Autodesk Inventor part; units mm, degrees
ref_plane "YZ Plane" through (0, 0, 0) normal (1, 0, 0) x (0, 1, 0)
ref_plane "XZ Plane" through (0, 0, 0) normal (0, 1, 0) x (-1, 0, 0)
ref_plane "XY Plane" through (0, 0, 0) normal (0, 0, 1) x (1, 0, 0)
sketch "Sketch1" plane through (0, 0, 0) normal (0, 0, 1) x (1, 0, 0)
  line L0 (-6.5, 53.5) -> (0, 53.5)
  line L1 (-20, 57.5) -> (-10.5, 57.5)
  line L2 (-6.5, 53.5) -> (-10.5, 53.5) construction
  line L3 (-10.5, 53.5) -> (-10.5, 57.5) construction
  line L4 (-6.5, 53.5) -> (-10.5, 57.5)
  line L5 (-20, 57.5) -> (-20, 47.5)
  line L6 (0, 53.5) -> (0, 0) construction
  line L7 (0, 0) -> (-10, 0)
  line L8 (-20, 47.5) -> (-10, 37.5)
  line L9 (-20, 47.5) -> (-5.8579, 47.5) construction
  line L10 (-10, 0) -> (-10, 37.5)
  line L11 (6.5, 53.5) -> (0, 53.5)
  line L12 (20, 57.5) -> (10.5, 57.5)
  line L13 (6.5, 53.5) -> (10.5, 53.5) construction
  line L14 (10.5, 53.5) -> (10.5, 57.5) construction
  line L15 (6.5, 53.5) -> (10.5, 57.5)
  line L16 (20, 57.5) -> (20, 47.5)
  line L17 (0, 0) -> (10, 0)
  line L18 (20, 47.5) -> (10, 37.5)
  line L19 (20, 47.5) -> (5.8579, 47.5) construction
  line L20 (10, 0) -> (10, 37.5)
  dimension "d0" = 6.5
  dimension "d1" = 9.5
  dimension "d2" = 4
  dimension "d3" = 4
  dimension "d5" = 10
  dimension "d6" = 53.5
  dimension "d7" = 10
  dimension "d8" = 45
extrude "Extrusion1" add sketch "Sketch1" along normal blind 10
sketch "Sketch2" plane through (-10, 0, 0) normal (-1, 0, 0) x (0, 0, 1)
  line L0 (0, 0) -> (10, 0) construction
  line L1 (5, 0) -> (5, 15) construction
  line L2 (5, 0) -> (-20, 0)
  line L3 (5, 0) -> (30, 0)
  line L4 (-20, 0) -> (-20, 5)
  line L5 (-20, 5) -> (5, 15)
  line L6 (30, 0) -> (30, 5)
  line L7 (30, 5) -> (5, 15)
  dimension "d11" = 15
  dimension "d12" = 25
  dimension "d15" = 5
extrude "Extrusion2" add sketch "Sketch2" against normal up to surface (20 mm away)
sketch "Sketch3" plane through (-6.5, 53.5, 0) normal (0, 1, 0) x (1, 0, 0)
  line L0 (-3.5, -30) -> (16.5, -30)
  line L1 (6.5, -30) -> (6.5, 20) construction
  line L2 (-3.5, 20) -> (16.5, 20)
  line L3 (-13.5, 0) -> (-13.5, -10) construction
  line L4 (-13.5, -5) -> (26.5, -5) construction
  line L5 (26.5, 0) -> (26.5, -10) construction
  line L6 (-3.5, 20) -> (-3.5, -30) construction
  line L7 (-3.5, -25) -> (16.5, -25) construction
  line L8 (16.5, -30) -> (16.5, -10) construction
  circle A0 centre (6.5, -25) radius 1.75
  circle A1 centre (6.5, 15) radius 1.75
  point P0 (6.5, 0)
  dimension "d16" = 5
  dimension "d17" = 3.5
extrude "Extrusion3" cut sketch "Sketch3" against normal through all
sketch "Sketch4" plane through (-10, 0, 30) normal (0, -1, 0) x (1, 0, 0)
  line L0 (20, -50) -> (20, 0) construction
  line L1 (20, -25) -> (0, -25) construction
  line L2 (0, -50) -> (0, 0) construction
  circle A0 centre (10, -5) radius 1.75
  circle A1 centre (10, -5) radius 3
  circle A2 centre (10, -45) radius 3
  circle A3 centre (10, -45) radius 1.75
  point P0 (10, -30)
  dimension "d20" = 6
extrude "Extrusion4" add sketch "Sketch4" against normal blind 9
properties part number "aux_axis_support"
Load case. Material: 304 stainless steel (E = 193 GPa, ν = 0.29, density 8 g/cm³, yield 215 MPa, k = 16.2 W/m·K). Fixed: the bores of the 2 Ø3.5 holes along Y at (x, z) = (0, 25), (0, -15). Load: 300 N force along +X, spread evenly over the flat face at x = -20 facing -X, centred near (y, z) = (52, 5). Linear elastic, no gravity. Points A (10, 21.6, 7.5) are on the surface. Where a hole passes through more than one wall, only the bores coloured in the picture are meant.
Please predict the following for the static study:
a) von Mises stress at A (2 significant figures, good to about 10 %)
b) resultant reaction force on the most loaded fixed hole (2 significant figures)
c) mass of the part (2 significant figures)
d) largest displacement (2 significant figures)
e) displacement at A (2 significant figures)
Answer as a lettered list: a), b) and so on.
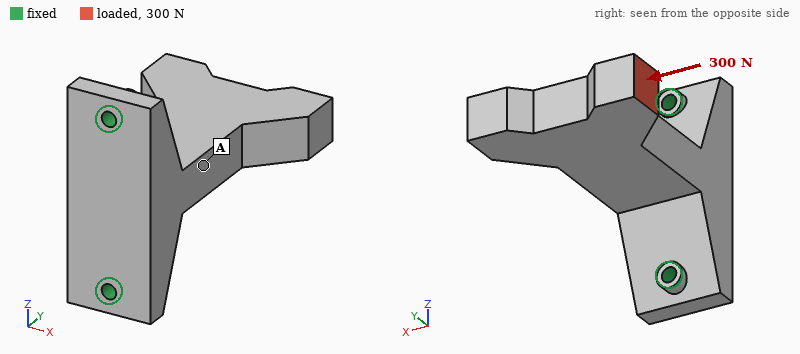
a) 14 MPa
b) 150 N
c) 170 g
d) 36 µm
e) 11 µm
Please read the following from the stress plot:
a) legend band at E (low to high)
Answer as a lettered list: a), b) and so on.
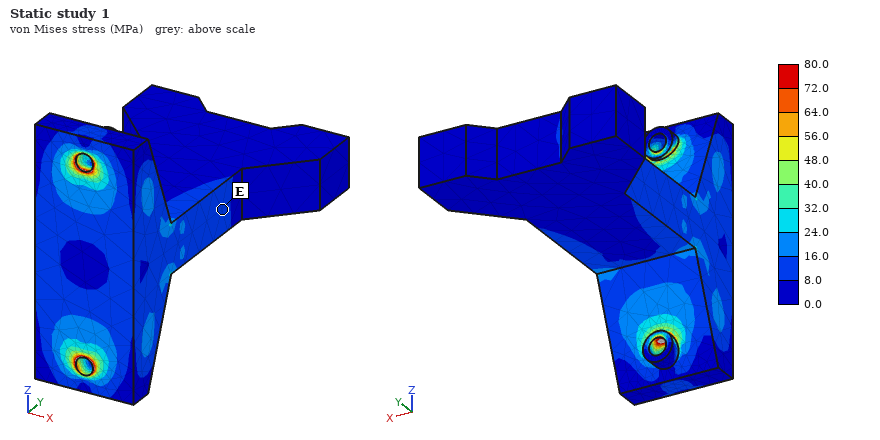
a) 8.0 to 16.0 MPa
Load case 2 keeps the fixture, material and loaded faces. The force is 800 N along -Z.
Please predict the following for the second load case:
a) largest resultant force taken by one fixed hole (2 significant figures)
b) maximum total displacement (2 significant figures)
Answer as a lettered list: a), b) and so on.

a) 1.3 kN
b) 0.12 mm
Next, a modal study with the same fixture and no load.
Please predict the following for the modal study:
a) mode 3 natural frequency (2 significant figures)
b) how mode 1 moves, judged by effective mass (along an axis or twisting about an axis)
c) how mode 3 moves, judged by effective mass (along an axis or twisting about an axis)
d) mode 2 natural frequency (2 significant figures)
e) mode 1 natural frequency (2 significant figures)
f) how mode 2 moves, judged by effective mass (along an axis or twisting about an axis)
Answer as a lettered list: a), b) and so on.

a) 6200 Hz
b) along X
c) twisting about Y
d) 2600 Hz
e) 2200 Hz
f) along Z
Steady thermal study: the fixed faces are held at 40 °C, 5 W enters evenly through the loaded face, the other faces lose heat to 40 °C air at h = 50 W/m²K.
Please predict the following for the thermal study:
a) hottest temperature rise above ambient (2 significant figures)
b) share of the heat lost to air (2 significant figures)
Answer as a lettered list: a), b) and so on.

a) 60 K
b) 77 %
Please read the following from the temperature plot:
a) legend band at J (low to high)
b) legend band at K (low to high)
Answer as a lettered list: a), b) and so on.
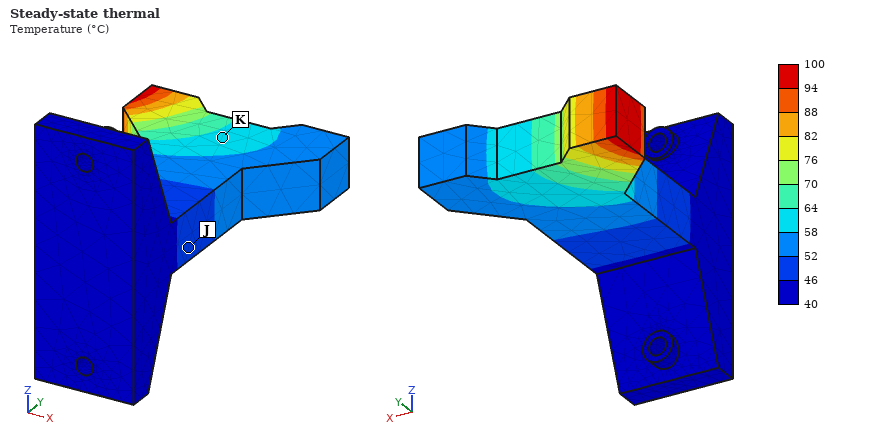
a) 46 to 52 °C
b) 58 to 64 °C
